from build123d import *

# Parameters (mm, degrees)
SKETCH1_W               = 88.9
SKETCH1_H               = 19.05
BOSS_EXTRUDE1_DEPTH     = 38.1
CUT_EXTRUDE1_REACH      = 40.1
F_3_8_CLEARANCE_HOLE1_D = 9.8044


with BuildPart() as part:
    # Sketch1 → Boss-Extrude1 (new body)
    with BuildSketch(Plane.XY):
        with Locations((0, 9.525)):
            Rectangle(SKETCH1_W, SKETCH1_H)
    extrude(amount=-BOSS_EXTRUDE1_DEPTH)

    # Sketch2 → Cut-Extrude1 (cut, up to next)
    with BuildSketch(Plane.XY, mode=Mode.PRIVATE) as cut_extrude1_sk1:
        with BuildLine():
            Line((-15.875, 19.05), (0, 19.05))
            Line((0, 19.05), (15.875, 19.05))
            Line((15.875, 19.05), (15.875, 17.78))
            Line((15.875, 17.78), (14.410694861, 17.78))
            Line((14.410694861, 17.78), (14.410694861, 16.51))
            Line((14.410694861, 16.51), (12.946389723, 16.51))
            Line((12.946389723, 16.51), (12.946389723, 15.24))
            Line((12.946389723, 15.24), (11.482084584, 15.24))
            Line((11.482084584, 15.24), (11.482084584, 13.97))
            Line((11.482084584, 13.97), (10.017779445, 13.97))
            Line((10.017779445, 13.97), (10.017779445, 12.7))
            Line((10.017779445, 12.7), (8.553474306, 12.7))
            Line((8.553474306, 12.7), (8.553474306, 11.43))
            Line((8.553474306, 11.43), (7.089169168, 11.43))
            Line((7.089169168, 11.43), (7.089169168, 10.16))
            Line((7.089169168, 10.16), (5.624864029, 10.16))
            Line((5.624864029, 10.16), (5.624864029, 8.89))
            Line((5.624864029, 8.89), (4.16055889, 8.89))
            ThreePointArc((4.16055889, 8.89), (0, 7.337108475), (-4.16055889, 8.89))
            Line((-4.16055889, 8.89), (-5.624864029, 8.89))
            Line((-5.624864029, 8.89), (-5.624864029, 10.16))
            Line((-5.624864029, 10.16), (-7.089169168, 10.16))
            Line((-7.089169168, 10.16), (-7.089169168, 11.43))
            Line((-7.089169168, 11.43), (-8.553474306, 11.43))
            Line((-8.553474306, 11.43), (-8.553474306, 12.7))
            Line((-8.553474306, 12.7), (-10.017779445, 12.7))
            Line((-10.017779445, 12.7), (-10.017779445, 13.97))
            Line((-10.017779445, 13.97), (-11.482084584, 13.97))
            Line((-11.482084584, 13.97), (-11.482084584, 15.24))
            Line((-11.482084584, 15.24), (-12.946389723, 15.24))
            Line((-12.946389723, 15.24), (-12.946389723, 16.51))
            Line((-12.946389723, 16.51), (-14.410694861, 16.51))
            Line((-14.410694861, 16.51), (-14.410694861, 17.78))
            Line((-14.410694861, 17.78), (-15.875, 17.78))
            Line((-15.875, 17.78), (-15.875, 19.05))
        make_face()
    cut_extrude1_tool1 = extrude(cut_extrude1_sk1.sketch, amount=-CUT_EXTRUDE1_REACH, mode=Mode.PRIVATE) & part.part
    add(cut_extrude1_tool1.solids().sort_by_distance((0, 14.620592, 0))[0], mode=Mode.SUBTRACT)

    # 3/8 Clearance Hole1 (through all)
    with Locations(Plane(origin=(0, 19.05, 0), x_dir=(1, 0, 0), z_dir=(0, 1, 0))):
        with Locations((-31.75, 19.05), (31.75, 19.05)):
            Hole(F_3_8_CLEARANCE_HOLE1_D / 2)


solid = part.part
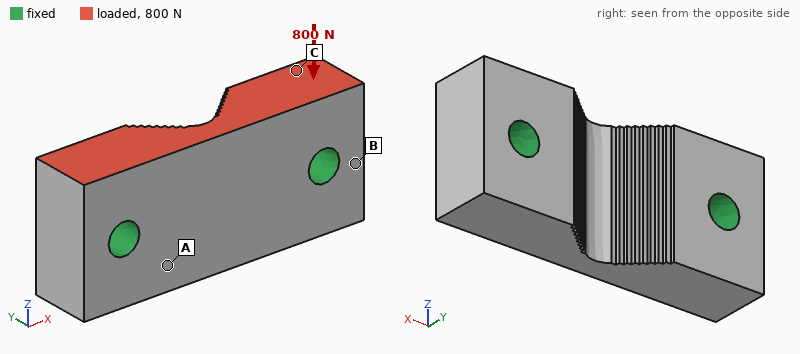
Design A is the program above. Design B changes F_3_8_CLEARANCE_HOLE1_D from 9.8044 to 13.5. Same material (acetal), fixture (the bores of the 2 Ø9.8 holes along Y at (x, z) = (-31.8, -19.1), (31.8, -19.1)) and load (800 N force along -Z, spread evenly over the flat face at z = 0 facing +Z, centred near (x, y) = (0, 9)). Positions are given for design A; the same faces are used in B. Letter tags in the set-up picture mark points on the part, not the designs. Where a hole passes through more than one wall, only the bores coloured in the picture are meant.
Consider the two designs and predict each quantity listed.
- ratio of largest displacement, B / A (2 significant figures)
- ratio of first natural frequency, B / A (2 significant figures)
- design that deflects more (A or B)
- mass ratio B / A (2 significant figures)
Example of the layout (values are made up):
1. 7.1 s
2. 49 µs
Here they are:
1. 0.81
2. 1.2
3. A
4. 0.95
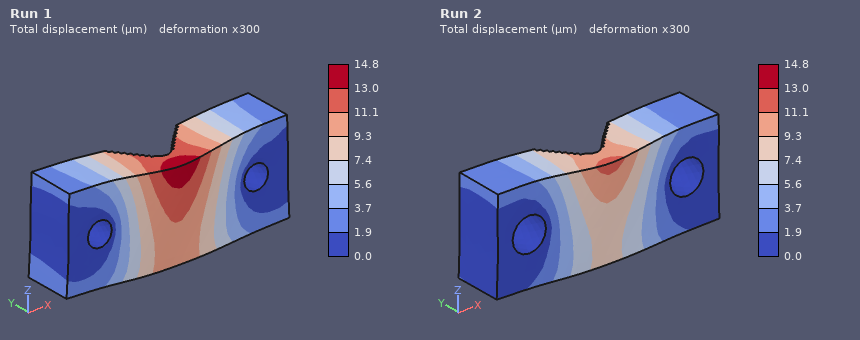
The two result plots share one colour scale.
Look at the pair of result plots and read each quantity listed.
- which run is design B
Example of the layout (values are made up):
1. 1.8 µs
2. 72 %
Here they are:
1. Run 2
